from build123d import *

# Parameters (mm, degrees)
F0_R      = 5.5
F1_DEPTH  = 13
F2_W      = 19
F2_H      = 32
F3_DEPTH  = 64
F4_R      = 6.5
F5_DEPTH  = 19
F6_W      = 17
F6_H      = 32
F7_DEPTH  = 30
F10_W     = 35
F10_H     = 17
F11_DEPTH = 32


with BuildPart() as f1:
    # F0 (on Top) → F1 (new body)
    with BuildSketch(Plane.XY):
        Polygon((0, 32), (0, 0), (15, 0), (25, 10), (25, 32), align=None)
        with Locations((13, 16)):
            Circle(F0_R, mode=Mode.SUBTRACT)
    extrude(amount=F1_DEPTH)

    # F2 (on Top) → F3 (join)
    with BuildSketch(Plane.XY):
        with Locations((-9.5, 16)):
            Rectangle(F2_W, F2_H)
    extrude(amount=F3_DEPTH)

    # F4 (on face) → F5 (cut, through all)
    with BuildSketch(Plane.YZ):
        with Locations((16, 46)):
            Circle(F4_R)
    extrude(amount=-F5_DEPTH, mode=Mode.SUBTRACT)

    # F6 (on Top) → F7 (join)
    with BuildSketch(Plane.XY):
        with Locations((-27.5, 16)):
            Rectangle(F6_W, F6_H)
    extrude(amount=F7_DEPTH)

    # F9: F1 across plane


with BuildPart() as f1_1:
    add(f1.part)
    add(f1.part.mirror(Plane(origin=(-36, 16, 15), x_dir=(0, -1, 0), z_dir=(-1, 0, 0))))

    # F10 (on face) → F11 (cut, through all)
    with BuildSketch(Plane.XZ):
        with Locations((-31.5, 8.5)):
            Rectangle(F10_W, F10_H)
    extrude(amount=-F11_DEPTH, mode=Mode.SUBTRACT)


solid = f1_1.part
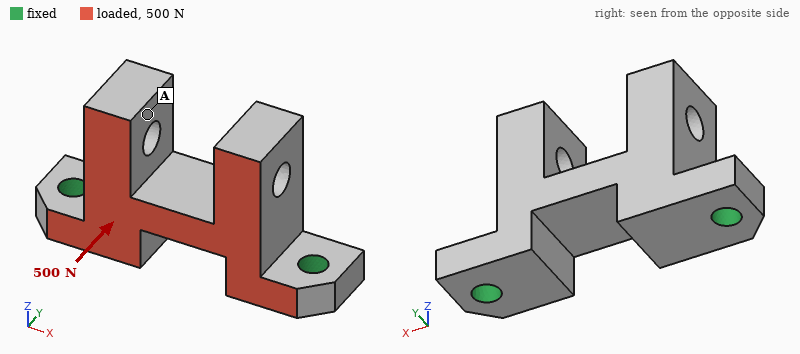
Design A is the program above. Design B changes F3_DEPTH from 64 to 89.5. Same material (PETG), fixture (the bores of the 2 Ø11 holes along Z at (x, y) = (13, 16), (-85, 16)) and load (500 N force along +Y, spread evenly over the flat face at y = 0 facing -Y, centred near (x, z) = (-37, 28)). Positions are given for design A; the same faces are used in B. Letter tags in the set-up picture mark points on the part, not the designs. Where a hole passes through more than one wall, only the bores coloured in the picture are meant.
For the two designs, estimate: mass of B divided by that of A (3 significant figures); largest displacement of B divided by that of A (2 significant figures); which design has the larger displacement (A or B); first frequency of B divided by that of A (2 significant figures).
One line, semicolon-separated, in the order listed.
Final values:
1.30; 2.1; B; 0.58
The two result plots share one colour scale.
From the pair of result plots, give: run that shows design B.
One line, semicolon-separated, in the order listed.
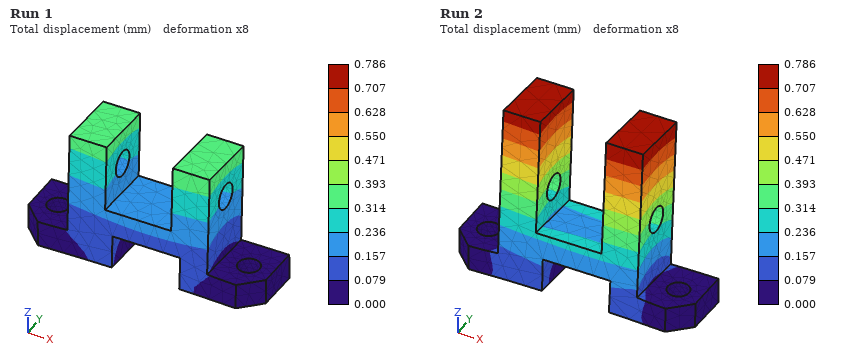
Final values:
Run 2
